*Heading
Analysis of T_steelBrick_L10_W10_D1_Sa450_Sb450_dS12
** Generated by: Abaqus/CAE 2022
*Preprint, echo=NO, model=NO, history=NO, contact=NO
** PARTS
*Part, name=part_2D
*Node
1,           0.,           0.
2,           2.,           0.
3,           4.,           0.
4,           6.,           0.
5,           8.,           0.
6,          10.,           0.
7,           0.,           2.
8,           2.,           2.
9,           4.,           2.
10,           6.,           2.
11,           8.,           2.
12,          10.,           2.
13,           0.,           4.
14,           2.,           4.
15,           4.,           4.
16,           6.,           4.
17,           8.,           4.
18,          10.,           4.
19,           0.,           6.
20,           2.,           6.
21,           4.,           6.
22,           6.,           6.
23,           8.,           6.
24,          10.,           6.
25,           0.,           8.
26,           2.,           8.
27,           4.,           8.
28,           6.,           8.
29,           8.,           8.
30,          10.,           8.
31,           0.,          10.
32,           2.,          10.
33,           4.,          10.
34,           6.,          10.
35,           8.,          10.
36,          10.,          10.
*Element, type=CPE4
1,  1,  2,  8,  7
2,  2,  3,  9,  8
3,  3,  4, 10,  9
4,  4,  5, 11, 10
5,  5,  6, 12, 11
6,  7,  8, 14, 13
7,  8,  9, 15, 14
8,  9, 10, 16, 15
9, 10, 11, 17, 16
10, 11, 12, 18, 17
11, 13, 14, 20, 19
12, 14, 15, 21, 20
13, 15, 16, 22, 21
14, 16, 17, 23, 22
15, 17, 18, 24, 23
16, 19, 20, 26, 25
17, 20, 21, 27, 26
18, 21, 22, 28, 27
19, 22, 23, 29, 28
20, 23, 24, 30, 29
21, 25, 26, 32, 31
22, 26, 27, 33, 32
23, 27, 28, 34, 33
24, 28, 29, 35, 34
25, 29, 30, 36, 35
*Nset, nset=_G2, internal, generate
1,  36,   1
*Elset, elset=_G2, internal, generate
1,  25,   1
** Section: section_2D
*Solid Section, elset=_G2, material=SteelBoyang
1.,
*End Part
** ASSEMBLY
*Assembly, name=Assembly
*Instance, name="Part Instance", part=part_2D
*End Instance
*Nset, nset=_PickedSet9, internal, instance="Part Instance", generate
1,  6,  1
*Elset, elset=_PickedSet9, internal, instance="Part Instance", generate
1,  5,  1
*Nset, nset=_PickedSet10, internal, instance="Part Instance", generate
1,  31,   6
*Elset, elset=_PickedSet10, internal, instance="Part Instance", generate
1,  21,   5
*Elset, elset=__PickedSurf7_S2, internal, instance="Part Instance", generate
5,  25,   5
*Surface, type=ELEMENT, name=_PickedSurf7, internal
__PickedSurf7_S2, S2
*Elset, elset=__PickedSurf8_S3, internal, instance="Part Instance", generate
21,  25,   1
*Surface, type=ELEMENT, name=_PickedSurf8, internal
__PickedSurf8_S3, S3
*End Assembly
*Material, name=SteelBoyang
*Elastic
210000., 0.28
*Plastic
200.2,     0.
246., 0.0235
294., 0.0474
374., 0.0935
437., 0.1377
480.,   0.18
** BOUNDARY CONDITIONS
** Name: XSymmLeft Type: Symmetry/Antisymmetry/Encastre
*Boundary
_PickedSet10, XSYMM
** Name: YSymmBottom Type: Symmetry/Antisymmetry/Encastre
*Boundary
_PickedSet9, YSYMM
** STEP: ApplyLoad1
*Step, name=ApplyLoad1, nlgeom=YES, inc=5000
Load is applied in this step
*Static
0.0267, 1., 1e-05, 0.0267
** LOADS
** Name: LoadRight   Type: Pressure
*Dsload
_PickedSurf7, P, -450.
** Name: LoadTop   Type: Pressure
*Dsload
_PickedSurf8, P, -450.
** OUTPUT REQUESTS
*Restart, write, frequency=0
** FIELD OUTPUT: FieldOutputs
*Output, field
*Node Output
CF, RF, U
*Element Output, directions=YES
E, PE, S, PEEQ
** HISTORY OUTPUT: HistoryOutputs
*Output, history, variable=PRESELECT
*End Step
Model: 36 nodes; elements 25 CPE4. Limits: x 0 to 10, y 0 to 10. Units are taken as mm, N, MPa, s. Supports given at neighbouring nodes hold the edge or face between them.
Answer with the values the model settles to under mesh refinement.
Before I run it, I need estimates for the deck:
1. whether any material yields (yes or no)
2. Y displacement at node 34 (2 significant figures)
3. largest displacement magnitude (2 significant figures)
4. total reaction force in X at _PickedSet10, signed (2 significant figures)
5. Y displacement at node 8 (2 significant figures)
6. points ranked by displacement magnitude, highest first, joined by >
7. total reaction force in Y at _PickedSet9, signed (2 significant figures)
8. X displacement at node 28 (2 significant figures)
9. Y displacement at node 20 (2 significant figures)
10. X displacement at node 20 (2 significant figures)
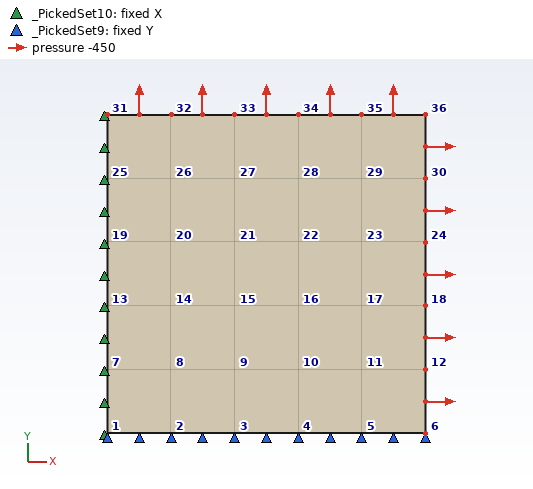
no
0.012 mm
0.017 mm
-4500 N
0.0024 mm
node 34 > node 28 > node 20 > node 8 > node 1
-4500 N
0.0072 mm
0.0072 mm
0.0024 mm
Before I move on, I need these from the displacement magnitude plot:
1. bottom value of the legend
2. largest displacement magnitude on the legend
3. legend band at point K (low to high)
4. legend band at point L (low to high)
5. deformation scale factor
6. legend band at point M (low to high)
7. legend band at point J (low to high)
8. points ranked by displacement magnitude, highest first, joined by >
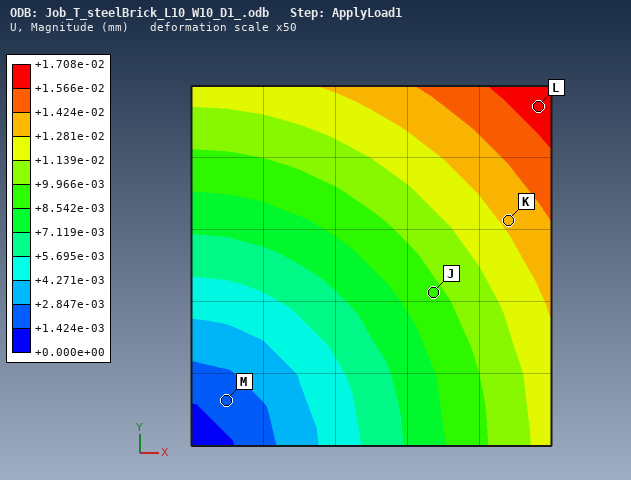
+0.000e+00 mm
+1.708e-02 mm
+1.281e-02 to +1.424e-02 mm
+1.566e-02 to +1.708e-02 mm
50
+1.424e-03 to +2.847e-03 mm
+8.542e-03 to +9.966e-03 mm
L > K > J > M
